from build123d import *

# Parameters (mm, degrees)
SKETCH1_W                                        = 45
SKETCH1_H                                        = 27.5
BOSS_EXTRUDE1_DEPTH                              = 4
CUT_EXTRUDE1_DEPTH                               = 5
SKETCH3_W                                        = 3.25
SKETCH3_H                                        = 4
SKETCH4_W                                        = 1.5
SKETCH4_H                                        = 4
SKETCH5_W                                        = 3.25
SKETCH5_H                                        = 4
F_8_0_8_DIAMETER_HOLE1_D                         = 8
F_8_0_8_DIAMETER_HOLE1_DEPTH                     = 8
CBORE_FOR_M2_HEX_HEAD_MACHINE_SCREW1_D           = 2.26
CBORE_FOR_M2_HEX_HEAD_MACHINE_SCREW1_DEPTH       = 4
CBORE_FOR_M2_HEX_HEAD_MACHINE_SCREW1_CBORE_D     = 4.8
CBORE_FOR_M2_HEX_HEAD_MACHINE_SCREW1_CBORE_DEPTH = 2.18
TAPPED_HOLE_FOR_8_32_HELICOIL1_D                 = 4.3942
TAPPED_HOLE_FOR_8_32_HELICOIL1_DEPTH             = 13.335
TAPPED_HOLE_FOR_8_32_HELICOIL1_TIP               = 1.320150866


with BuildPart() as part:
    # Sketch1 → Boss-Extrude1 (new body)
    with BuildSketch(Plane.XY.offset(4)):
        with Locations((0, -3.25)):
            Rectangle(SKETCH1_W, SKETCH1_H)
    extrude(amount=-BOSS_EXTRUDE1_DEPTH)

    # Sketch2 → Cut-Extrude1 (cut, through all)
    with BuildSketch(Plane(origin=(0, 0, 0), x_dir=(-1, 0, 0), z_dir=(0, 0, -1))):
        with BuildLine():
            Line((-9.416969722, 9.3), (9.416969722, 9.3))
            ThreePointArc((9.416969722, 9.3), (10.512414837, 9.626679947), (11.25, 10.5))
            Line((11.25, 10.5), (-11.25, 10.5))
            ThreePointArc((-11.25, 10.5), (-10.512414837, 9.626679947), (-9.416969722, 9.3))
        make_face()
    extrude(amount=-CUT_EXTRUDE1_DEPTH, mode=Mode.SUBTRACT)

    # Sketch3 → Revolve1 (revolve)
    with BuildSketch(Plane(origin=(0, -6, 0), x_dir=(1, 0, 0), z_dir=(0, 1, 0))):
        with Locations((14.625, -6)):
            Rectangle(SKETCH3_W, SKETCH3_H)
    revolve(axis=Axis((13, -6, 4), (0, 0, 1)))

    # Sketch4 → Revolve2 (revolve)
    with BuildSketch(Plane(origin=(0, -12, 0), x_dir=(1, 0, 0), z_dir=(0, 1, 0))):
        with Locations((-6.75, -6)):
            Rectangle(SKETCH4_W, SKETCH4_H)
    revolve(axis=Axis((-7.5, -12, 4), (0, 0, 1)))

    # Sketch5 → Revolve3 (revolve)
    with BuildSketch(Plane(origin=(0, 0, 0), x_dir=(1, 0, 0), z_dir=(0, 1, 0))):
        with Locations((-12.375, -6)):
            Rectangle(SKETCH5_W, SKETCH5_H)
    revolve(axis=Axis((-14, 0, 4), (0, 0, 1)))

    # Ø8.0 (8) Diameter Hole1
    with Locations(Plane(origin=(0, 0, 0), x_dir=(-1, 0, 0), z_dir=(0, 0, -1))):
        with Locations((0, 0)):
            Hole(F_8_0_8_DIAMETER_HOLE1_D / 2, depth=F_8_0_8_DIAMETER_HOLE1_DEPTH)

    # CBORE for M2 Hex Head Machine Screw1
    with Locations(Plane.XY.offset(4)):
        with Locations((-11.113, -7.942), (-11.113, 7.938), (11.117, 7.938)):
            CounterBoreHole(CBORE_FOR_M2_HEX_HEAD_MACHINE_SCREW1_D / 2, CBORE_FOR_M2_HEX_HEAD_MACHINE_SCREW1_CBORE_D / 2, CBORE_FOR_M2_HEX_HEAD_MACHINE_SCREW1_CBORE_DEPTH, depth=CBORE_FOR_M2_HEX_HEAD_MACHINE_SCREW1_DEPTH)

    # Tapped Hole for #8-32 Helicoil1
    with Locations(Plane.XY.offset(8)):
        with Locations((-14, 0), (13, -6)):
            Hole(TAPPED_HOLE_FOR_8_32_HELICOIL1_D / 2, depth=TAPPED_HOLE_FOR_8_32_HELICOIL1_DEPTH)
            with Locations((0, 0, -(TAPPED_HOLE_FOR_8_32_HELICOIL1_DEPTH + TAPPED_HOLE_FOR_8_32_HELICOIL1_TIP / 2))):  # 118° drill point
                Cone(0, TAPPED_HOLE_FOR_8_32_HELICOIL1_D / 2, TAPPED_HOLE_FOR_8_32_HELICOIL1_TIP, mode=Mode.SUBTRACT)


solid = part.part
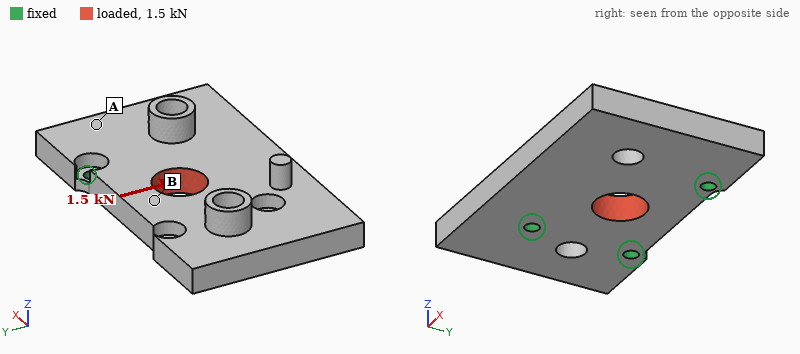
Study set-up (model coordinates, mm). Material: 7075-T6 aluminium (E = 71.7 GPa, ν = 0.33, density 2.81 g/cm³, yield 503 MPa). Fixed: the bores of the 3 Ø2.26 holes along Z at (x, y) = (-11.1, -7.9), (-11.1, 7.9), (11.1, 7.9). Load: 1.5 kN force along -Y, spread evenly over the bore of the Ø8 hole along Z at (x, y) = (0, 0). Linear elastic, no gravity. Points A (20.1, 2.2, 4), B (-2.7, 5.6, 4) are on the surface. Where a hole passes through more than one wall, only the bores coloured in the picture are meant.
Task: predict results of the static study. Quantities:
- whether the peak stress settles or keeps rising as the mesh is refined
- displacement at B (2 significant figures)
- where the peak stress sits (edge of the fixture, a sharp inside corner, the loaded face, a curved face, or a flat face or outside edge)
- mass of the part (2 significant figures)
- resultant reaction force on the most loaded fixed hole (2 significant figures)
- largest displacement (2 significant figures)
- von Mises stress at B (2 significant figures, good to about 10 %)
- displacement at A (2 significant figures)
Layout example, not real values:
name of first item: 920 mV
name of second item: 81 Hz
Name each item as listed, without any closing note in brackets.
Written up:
whether the peak stress settles or keeps rising as the mesh is refined: keeps rising
displacement at B: 6.4 µm
where the peak stress sits: edge of the fixture
mass of the part: 13 g
resultant reaction force on the most loaded fixed hole: 620 N
largest displacement: 20 µm
von Mises stress at B: 26 MPa
displacement at A: 8.4 µm
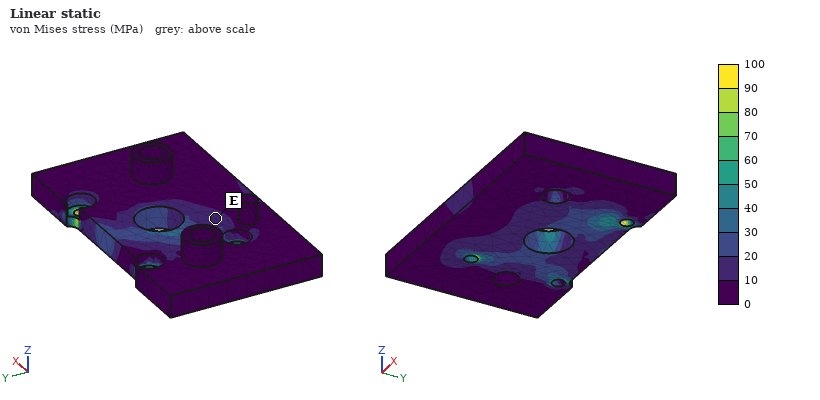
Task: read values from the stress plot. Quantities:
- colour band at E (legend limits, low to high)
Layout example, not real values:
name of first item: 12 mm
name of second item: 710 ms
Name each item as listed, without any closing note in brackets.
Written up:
colour band at E: 10 to 20 MPa
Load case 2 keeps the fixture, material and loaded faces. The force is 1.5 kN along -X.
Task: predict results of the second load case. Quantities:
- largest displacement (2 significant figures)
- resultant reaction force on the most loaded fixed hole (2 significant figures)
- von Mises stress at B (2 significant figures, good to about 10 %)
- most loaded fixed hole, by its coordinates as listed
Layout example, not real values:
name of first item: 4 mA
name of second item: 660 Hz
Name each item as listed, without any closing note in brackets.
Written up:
largest displacement: 13 µm
resultant reaction force on the most loaded fixed hole: 610 N
von Mises stress at B: 15 MPa
most loaded fixed hole, by its coordinates as listed: (-11.1, -7.9)
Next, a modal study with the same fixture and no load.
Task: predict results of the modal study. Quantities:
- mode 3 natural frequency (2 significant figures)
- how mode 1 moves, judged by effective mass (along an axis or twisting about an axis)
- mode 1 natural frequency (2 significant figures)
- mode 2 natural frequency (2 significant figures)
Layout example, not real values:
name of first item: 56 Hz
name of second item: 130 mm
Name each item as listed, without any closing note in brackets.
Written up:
mode 3 natural frequency: 15 kHz
how mode 1 moves, judged by effective mass: along Z
mode 1 natural frequency: 4400 Hz
mode 2 natural frequency: 12 kHz
